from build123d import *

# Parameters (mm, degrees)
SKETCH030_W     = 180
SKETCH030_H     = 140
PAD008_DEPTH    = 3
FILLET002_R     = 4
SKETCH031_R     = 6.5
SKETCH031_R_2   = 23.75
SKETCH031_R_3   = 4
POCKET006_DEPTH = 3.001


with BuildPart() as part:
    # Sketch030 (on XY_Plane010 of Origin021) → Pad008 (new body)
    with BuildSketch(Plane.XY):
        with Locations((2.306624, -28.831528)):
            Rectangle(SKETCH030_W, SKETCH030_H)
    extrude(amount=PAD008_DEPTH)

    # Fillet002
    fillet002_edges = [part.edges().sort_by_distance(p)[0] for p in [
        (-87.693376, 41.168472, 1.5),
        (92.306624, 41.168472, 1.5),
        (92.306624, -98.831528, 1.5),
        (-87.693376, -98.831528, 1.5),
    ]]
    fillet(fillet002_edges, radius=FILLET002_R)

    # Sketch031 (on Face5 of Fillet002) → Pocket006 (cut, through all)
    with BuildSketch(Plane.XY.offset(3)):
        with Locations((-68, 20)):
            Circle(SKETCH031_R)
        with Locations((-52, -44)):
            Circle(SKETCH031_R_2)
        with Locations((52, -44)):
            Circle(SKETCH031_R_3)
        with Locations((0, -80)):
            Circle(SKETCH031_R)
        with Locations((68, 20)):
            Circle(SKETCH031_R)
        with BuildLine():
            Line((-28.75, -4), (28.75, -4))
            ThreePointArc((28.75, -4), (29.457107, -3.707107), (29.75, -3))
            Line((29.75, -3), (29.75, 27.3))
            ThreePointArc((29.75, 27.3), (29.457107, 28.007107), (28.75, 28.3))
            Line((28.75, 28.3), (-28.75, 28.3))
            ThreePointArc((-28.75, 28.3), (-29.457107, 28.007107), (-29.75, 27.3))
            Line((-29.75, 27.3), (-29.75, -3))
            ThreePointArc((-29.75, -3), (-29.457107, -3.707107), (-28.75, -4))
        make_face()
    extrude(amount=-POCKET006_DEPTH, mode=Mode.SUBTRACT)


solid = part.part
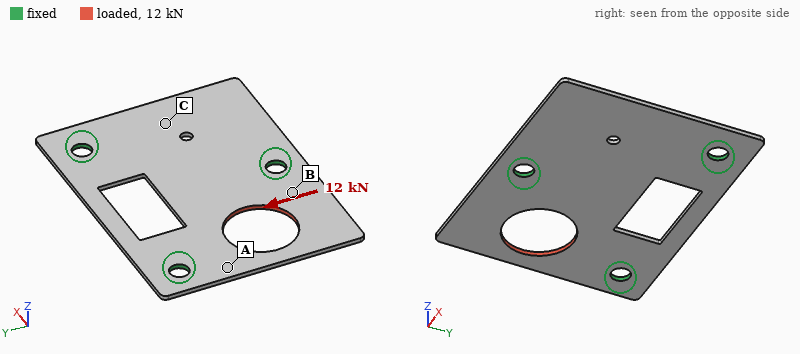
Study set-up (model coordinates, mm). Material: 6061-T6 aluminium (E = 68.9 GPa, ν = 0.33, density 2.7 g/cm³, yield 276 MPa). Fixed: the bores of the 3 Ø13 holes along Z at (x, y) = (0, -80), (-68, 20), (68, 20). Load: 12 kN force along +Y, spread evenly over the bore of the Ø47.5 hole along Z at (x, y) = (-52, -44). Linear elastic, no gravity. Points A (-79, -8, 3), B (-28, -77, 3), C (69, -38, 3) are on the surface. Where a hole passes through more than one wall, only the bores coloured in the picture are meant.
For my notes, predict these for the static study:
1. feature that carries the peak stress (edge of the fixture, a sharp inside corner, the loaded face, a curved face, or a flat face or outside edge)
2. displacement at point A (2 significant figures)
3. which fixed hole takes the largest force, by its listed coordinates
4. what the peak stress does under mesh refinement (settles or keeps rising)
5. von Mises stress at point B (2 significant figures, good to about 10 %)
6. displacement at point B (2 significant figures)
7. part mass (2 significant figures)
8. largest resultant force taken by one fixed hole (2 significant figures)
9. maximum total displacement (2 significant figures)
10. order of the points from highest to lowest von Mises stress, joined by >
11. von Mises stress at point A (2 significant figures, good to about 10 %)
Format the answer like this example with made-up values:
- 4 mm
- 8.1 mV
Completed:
- edge of the fixture
- 27 µm
- (-68, 20)
- keeps rising
- 37 MPa
- 40 µm
- 170 g
- 7.1 kN
- 91 µm
- A > B > C
- 71 MPa
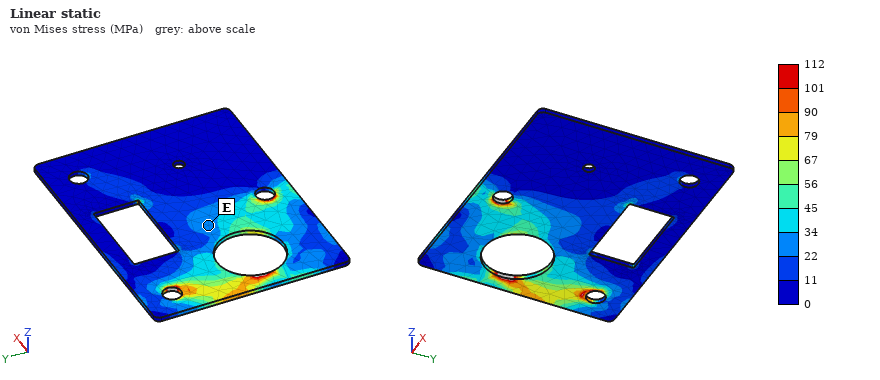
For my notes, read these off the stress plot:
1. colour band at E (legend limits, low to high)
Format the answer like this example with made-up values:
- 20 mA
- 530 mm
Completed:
- 22 to 34 MPa
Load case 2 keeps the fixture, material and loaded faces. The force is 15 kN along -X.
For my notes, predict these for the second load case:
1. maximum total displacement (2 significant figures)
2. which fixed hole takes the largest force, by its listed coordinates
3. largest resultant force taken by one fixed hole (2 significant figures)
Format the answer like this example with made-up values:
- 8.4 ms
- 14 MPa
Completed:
- 0.15 mm
- (0, -80)
- 9.2 kN
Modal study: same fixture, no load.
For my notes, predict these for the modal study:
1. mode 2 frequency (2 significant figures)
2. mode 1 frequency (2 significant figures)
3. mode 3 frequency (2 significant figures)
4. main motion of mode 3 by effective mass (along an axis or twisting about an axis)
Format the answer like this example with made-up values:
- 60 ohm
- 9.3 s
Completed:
- 510 Hz
- 490 Hz
- 1100 Hz
- along Z
